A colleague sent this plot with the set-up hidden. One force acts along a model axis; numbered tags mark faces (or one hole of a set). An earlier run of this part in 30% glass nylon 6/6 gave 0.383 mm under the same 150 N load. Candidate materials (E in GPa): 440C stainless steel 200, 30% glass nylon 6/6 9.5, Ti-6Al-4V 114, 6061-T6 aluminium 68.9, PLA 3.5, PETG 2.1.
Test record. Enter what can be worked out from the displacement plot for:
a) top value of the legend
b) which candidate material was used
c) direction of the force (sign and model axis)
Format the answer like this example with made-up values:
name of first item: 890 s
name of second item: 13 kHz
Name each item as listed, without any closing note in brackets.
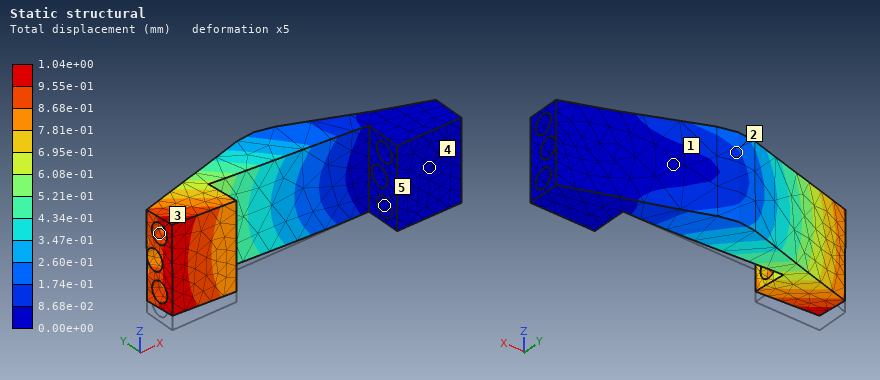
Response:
top value of the legend: 1.04e+00 mm
which candidate material was used: PLA
direction of the force: +Z
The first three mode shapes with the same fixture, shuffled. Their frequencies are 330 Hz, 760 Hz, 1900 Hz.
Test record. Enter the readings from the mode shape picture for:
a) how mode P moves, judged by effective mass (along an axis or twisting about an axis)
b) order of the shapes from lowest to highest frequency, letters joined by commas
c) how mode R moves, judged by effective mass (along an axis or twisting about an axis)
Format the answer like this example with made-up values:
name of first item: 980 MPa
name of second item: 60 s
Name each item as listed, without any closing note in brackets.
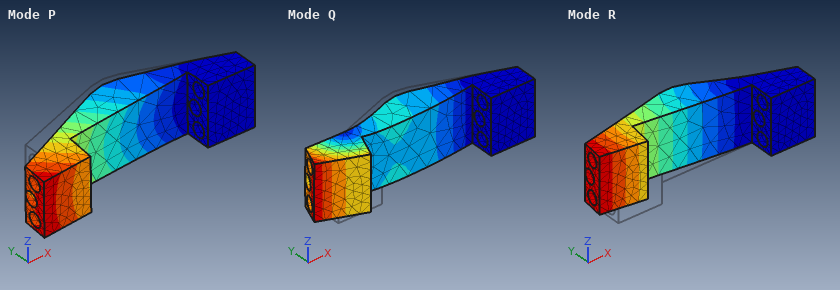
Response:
how mode P moves, judged by effective mass: along Z
order of the shapes from lowest to highest frequency, letters joined by commas: R, P, Q
how mode R moves, judged by effective mass: along Y
